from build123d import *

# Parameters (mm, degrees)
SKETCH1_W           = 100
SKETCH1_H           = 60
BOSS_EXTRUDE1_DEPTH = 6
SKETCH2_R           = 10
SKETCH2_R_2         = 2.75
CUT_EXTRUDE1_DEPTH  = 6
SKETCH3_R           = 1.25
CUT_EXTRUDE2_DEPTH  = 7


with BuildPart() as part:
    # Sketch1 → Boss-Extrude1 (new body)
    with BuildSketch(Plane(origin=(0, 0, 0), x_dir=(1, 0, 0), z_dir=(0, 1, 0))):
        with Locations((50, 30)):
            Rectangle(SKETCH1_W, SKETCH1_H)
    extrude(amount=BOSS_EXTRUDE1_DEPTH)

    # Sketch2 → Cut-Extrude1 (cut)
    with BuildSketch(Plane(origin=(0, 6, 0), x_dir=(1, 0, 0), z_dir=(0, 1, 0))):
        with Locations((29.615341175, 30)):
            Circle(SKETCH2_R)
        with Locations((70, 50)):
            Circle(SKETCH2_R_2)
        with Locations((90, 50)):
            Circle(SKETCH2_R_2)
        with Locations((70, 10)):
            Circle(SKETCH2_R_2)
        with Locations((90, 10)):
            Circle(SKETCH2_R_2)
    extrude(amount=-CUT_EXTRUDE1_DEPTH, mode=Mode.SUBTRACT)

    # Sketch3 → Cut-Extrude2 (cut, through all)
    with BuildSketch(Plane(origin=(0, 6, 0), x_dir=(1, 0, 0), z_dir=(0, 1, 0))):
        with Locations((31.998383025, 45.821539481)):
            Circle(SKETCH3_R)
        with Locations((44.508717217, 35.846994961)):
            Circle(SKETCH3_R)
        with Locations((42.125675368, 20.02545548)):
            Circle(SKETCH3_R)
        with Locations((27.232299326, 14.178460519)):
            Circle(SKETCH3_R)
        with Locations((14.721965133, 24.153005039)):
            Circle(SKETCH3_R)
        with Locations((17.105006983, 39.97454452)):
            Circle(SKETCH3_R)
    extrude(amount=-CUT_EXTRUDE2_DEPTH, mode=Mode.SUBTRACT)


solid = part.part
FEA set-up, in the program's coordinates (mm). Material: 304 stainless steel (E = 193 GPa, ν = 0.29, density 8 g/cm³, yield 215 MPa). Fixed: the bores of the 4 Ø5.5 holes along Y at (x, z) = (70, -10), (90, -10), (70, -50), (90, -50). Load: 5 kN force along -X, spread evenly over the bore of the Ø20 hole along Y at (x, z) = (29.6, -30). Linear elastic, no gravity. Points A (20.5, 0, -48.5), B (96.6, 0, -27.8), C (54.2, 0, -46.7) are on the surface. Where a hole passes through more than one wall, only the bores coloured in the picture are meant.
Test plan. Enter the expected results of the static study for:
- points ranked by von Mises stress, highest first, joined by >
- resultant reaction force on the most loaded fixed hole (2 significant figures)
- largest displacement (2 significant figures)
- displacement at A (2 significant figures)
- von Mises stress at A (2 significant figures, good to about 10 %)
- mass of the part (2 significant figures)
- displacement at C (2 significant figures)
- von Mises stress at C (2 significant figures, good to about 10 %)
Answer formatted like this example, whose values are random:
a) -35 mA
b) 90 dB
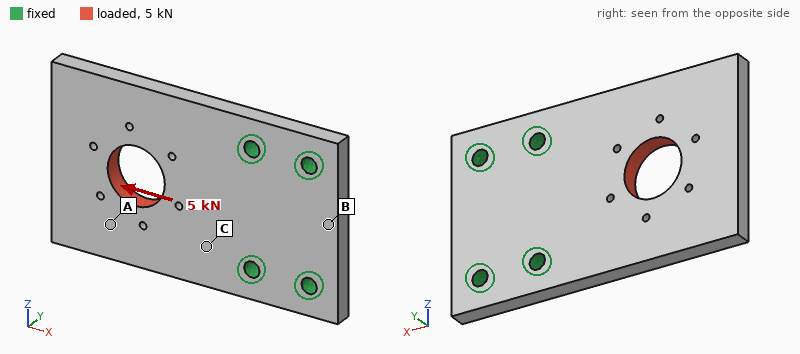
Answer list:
a) C > A > B
b) 2.0 kN
c) 5.9 µm
d) 3.6 µm
e) 8.4 MPa
f) 270 g
g) 1.5 µm
h) 17 MPa
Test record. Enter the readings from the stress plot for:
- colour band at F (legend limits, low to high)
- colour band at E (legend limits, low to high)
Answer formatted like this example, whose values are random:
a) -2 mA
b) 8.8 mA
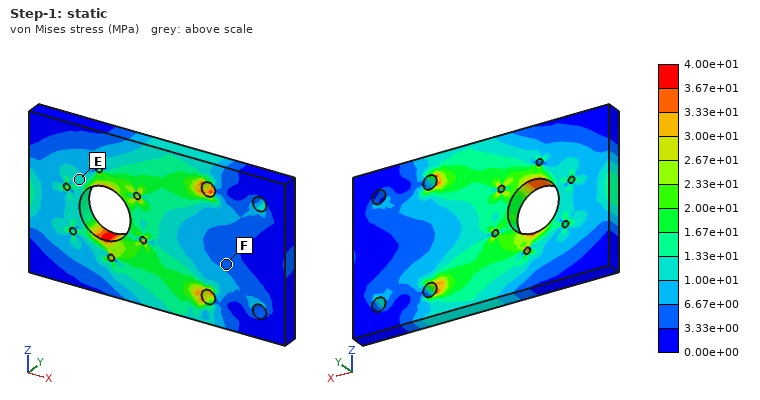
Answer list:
a) 3.33e+00 to 6.67e+00 MPa
b) 1.00e+01 to 1.33e+01 MPa
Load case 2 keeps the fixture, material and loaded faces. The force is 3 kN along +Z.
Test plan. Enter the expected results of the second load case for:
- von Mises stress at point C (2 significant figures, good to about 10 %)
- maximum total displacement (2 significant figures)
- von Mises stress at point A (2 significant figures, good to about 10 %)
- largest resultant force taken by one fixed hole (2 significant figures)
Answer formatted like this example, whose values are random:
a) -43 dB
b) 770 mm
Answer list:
a) 17 MPa
b) 17 µm
c) 5.0 MPa
d) 2.8 kN
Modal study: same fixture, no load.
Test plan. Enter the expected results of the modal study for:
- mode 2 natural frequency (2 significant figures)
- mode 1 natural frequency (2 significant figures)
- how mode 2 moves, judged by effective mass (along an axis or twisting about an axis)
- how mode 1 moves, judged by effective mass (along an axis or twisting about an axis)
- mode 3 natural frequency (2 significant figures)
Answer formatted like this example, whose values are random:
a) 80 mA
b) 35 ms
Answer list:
a) 2500 Hz
b) 960 Hz
c) twisting about X
d) along Y
e) 5500 Hz
